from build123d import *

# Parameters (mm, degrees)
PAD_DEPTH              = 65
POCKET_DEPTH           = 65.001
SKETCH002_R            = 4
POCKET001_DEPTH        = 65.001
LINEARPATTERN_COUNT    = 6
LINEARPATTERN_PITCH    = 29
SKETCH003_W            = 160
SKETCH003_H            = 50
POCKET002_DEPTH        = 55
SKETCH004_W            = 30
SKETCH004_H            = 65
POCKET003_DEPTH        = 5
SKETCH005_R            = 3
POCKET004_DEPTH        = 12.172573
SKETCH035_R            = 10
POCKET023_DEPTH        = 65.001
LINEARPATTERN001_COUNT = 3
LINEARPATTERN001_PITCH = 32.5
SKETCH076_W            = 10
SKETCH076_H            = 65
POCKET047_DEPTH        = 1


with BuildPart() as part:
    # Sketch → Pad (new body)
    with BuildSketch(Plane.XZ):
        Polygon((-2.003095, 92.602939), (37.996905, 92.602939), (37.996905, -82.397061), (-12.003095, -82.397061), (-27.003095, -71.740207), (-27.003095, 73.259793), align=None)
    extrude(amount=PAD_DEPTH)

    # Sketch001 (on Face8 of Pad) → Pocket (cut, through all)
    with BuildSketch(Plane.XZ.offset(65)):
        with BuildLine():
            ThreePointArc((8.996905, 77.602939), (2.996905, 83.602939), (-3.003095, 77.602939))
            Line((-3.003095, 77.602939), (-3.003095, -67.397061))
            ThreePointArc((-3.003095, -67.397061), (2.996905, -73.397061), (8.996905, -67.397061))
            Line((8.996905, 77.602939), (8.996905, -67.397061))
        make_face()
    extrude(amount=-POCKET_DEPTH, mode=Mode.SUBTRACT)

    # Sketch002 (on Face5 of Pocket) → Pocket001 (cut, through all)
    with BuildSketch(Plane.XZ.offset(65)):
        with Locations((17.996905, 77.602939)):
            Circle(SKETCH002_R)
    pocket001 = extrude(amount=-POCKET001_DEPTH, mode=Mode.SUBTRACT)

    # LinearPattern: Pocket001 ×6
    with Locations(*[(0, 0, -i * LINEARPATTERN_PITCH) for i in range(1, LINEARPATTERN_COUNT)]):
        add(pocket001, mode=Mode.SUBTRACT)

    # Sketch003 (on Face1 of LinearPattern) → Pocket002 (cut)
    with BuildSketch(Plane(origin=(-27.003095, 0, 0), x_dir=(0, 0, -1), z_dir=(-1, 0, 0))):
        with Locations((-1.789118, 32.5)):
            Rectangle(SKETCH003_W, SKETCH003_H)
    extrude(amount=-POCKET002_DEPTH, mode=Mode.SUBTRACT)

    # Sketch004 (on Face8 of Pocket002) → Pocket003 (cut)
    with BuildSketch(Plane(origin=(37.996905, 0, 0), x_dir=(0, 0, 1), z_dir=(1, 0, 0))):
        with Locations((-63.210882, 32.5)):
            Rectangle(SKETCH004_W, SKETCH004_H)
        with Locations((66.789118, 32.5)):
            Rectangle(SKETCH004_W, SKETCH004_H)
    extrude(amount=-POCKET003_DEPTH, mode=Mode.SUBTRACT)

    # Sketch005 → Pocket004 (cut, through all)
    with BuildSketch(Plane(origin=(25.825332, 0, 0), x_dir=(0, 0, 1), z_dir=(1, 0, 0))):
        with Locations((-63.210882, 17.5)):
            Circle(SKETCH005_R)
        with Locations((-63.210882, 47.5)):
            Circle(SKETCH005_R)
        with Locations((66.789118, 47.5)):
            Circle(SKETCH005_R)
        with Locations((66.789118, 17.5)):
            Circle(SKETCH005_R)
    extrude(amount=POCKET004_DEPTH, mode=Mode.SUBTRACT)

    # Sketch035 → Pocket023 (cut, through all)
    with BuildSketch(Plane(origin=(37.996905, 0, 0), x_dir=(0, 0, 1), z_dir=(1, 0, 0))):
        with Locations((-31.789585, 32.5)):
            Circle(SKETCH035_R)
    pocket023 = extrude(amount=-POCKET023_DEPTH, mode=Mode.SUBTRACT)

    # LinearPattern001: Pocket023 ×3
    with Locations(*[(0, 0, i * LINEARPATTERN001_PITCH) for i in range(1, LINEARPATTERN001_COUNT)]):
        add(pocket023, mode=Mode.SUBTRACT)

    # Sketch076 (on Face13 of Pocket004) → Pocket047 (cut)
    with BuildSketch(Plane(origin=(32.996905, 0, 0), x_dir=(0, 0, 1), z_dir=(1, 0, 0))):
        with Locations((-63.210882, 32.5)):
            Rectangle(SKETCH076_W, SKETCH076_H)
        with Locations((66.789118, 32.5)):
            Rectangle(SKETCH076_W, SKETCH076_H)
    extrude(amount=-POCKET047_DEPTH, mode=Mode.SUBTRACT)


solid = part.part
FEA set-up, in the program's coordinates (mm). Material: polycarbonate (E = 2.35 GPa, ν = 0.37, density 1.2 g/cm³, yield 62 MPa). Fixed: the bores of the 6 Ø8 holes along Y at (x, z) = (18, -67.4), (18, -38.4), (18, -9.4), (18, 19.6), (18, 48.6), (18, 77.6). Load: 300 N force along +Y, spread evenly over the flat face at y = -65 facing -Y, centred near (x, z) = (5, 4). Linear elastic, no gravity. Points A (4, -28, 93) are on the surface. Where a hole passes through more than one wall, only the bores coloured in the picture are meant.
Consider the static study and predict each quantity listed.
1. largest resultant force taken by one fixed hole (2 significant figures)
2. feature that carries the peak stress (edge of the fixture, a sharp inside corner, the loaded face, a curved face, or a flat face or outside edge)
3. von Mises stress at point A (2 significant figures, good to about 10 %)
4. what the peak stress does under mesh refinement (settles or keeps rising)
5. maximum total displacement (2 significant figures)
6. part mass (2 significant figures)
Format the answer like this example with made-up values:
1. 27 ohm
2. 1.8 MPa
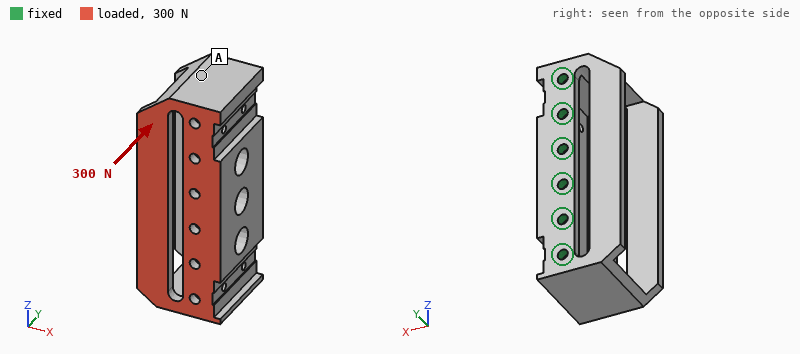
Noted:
1. 150 N
2. edge of the fixture
3. 1.1 MPa
4. keeps rising
5. 1.9 mm
6. 260 g
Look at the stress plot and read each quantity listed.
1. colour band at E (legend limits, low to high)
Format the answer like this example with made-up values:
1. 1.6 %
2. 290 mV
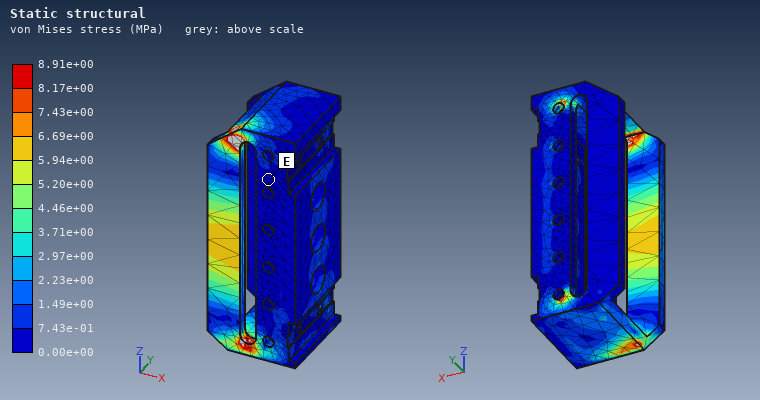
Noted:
1. 0.00e+00 to 7.43e-01 MPa
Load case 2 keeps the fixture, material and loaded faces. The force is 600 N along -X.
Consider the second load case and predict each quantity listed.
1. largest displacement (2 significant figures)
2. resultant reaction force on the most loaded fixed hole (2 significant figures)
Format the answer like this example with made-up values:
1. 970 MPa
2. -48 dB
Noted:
1. 2.4 mm
2. 410 N
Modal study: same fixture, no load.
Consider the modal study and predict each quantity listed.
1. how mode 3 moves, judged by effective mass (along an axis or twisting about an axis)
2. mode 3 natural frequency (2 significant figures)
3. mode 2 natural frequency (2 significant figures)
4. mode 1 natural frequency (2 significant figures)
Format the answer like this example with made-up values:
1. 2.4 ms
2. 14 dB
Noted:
1. along X
2. 350 Hz
3. 280 Hz
4. 250 Hz
